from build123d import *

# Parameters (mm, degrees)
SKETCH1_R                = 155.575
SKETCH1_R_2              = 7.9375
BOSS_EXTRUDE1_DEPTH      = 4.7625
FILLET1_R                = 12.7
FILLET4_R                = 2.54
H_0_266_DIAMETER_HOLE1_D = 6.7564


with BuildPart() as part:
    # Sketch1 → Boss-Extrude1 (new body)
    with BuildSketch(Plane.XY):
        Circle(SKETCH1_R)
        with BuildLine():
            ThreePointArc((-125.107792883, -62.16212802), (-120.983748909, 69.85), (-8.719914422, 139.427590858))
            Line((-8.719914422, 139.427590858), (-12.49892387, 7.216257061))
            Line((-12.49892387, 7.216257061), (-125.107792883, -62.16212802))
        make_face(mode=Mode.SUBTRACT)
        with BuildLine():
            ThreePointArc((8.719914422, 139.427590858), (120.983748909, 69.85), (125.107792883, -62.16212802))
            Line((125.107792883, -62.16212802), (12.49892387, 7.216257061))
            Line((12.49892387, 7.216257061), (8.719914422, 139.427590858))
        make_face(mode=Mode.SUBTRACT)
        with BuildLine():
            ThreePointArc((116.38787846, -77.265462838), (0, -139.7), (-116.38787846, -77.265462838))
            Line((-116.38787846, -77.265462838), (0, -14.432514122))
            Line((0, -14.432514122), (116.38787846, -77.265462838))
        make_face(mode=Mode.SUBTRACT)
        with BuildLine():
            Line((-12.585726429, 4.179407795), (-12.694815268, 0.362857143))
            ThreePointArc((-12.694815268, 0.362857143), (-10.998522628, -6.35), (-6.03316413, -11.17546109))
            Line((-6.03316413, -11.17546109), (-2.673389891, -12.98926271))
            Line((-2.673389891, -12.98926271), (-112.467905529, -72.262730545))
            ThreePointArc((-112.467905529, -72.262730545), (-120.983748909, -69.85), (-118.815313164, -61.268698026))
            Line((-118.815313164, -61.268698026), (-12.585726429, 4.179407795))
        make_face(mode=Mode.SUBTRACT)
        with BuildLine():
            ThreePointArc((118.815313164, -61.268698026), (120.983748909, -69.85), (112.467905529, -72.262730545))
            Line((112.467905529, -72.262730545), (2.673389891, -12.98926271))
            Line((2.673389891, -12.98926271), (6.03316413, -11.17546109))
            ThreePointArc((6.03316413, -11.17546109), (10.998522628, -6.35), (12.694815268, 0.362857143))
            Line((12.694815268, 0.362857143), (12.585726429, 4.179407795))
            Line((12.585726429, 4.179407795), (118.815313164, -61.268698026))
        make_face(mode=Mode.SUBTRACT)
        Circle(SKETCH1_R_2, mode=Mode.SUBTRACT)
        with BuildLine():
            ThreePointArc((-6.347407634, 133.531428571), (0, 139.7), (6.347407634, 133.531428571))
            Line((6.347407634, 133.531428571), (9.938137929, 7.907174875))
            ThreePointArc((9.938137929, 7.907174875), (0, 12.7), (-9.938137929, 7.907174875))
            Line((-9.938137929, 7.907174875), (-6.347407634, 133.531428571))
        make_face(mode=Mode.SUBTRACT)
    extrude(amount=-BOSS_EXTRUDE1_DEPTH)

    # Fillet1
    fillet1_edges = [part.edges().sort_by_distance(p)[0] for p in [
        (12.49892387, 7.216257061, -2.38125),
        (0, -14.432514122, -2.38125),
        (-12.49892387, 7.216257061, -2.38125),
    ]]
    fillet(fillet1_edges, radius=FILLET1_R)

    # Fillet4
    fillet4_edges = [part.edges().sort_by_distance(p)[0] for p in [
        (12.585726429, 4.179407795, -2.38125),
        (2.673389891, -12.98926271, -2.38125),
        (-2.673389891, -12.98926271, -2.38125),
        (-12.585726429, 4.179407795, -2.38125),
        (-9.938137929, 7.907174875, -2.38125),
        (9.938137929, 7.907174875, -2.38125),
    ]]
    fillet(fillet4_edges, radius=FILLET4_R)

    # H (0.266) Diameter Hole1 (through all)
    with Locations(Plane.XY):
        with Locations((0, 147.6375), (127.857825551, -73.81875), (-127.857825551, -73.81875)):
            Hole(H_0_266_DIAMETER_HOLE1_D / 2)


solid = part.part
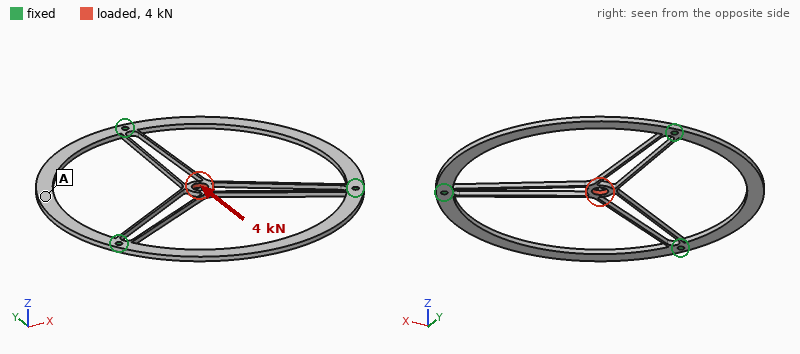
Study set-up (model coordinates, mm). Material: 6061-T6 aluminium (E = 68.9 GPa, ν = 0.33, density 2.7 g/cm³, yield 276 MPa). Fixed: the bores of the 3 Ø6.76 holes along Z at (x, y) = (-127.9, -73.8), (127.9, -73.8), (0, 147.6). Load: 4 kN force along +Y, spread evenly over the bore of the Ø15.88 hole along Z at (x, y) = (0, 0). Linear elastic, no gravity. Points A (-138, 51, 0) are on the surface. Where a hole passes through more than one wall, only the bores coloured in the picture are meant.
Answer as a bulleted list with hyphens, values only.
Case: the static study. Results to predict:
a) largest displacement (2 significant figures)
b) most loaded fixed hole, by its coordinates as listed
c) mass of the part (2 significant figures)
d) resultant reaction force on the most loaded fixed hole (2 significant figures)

- 0.23 mm
- (0, 147.6)
- 220 g
- 2.6 kN
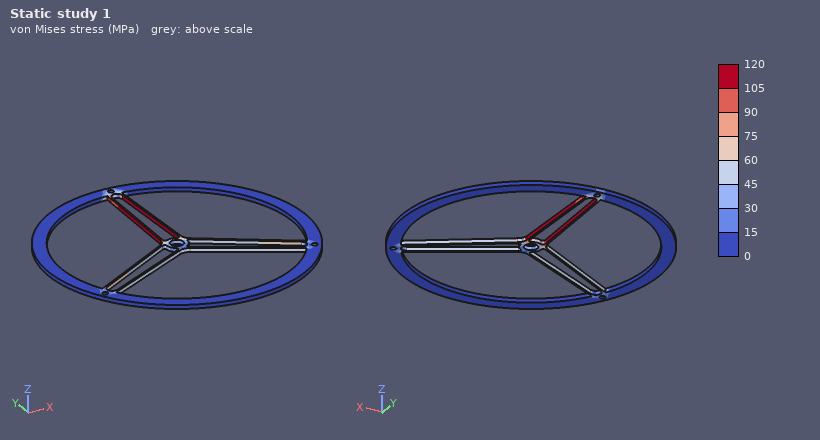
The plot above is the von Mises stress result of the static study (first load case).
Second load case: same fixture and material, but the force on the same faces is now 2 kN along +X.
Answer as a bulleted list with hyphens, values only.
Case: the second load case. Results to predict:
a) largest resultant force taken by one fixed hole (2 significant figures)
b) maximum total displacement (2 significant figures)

- 1.1 kN
- 0.11 mm
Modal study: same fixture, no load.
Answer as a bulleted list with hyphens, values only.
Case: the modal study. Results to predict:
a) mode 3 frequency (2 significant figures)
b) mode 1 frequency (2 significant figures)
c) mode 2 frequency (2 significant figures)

- 240 Hz
- 240 Hz
- 240 Hz
